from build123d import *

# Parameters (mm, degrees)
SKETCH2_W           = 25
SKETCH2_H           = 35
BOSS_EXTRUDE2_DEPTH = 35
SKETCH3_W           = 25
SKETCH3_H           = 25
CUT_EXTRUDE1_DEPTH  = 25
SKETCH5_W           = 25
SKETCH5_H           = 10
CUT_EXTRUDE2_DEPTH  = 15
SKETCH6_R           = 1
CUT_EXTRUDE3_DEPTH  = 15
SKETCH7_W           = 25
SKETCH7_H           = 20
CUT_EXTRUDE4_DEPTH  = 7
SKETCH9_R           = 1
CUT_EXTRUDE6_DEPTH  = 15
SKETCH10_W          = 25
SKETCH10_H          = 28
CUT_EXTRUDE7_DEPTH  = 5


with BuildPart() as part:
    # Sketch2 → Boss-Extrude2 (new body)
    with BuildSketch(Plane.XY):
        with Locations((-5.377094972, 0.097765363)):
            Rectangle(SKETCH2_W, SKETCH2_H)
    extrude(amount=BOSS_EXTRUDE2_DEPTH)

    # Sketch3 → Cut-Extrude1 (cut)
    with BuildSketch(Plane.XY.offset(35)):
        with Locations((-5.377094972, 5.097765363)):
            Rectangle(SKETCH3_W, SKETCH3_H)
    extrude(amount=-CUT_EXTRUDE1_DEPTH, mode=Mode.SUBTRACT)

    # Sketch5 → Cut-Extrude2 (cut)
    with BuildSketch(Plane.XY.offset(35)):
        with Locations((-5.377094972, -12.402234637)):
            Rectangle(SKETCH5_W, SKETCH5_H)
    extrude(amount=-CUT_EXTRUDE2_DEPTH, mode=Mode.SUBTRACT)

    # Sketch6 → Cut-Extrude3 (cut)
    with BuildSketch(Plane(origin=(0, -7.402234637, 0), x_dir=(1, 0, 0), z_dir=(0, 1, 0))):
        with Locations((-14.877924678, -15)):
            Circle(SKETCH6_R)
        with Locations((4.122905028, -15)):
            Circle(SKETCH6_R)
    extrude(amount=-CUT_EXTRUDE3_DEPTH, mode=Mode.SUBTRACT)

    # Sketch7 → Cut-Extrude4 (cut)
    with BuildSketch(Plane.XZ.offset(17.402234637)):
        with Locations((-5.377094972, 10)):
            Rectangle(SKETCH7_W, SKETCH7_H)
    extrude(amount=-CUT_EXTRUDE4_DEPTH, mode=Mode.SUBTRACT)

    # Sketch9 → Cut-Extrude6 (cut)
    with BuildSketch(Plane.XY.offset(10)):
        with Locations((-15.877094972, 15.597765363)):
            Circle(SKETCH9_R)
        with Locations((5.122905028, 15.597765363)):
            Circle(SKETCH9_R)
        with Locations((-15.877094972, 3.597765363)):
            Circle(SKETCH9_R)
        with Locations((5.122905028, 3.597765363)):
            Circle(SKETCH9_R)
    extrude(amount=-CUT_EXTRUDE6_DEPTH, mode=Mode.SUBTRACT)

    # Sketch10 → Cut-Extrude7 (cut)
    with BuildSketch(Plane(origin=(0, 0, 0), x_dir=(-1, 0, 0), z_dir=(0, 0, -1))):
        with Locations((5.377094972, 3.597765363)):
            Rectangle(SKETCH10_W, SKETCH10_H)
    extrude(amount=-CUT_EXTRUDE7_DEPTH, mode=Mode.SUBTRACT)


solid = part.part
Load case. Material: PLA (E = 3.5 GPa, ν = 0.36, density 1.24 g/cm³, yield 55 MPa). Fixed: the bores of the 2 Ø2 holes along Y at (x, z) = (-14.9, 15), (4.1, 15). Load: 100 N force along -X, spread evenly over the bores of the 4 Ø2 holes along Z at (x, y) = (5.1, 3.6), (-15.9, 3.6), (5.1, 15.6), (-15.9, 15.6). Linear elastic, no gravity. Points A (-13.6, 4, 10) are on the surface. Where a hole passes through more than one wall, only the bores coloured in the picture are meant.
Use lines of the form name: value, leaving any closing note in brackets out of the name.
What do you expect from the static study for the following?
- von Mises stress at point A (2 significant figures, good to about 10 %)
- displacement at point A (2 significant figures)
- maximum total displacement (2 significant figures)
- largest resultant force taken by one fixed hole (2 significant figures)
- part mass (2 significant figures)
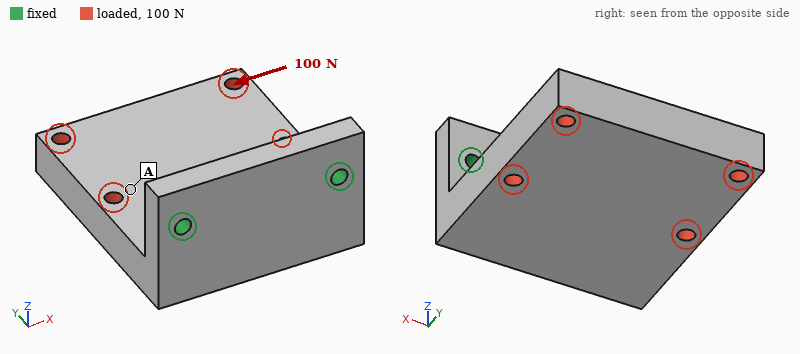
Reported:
von Mises stress at point A: 3.6 MPa
displacement at point A: 0.14 mm
maximum total displacement: 0.27 mm
largest resultant force taken by one fixed hole: 110 N
part mass: 5.2 g
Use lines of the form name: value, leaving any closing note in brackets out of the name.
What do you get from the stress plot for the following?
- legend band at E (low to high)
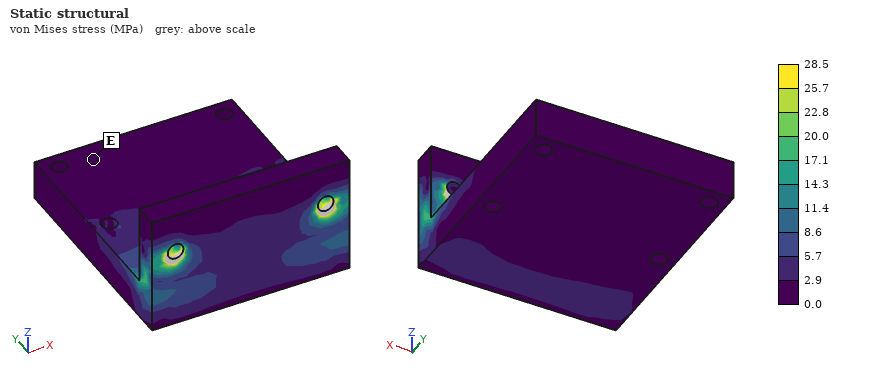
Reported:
legend band at E: 0.0 to 2.9 MPa
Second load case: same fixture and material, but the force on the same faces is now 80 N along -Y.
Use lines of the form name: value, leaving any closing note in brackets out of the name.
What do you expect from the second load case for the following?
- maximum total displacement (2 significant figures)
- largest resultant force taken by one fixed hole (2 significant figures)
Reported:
maximum total displacement: 0.39 mm
largest resultant force taken by one fixed hole: 40 N
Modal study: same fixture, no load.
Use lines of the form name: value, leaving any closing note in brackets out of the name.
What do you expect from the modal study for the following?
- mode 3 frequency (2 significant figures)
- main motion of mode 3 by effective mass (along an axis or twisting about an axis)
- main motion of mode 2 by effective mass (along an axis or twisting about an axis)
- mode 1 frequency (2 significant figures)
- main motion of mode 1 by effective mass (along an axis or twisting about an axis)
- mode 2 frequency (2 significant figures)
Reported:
mode 3 frequency: 4000 Hz
main motion of mode 3 by effective mass: along Y
main motion of mode 2 by effective mass: along X
mode 1 frequency: 770 Hz
main motion of mode 1 by effective mass: along Z
mode 2 frequency: 2100 Hz
